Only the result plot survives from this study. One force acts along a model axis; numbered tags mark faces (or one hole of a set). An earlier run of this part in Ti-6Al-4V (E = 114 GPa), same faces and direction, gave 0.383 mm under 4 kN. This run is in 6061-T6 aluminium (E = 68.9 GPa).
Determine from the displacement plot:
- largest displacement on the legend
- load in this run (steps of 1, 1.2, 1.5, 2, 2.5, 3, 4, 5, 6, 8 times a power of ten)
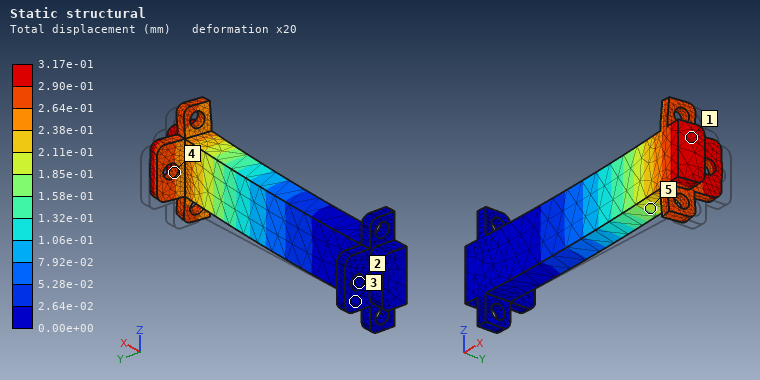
3.17e-01 mm
2 kN
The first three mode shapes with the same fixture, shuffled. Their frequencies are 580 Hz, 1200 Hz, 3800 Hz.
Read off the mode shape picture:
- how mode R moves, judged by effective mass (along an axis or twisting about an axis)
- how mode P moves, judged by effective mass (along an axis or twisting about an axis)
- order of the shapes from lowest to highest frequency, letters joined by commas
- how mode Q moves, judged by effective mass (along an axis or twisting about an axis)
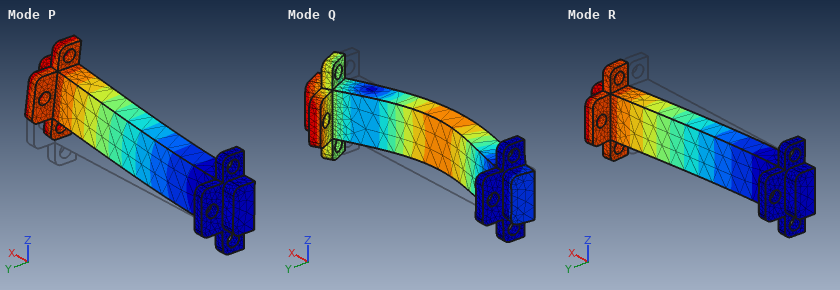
along Y
along Z
R, P, Q
along Y
